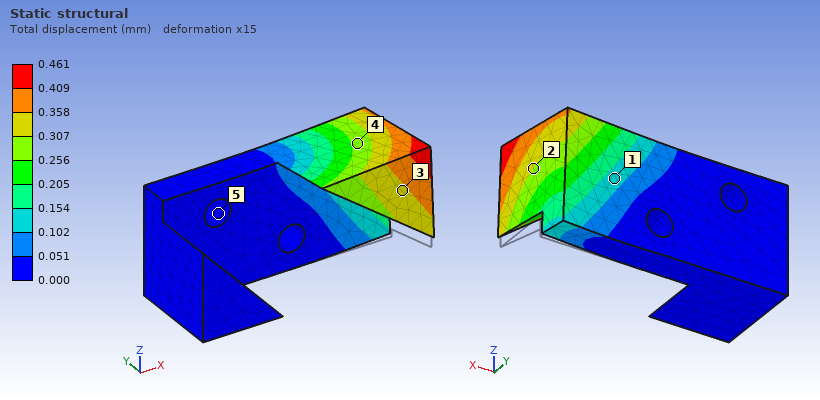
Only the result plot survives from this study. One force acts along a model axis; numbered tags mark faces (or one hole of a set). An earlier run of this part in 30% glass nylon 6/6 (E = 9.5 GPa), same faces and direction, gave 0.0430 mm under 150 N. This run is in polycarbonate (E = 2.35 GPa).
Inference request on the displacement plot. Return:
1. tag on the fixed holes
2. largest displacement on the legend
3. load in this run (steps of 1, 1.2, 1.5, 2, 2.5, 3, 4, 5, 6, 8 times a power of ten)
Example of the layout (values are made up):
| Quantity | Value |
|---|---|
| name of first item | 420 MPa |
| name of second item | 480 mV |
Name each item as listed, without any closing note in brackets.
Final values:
| Quantity | Value |
|---|---|
| tag on the fixed holes | 5 |
| largest displacement on the legend | 0.461 mm |
| load in this run | 400 N |
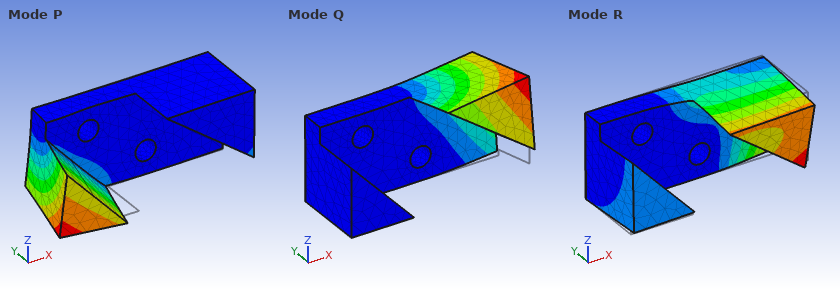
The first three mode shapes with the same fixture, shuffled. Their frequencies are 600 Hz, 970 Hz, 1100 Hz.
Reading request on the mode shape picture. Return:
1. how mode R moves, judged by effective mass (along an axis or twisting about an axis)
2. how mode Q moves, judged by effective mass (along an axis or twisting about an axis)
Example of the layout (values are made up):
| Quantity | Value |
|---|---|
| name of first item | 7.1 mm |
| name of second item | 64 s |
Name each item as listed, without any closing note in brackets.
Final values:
| Quantity | Value |
|---|---|
| how mode R moves, judged by effective mass | along Z |
| how mode Q moves, judged by effective mass | along Y |
